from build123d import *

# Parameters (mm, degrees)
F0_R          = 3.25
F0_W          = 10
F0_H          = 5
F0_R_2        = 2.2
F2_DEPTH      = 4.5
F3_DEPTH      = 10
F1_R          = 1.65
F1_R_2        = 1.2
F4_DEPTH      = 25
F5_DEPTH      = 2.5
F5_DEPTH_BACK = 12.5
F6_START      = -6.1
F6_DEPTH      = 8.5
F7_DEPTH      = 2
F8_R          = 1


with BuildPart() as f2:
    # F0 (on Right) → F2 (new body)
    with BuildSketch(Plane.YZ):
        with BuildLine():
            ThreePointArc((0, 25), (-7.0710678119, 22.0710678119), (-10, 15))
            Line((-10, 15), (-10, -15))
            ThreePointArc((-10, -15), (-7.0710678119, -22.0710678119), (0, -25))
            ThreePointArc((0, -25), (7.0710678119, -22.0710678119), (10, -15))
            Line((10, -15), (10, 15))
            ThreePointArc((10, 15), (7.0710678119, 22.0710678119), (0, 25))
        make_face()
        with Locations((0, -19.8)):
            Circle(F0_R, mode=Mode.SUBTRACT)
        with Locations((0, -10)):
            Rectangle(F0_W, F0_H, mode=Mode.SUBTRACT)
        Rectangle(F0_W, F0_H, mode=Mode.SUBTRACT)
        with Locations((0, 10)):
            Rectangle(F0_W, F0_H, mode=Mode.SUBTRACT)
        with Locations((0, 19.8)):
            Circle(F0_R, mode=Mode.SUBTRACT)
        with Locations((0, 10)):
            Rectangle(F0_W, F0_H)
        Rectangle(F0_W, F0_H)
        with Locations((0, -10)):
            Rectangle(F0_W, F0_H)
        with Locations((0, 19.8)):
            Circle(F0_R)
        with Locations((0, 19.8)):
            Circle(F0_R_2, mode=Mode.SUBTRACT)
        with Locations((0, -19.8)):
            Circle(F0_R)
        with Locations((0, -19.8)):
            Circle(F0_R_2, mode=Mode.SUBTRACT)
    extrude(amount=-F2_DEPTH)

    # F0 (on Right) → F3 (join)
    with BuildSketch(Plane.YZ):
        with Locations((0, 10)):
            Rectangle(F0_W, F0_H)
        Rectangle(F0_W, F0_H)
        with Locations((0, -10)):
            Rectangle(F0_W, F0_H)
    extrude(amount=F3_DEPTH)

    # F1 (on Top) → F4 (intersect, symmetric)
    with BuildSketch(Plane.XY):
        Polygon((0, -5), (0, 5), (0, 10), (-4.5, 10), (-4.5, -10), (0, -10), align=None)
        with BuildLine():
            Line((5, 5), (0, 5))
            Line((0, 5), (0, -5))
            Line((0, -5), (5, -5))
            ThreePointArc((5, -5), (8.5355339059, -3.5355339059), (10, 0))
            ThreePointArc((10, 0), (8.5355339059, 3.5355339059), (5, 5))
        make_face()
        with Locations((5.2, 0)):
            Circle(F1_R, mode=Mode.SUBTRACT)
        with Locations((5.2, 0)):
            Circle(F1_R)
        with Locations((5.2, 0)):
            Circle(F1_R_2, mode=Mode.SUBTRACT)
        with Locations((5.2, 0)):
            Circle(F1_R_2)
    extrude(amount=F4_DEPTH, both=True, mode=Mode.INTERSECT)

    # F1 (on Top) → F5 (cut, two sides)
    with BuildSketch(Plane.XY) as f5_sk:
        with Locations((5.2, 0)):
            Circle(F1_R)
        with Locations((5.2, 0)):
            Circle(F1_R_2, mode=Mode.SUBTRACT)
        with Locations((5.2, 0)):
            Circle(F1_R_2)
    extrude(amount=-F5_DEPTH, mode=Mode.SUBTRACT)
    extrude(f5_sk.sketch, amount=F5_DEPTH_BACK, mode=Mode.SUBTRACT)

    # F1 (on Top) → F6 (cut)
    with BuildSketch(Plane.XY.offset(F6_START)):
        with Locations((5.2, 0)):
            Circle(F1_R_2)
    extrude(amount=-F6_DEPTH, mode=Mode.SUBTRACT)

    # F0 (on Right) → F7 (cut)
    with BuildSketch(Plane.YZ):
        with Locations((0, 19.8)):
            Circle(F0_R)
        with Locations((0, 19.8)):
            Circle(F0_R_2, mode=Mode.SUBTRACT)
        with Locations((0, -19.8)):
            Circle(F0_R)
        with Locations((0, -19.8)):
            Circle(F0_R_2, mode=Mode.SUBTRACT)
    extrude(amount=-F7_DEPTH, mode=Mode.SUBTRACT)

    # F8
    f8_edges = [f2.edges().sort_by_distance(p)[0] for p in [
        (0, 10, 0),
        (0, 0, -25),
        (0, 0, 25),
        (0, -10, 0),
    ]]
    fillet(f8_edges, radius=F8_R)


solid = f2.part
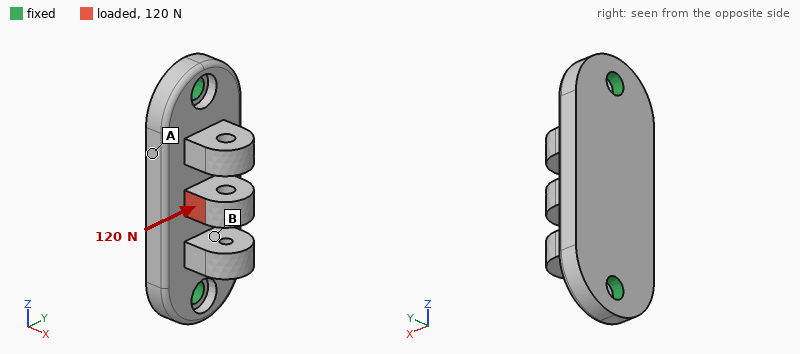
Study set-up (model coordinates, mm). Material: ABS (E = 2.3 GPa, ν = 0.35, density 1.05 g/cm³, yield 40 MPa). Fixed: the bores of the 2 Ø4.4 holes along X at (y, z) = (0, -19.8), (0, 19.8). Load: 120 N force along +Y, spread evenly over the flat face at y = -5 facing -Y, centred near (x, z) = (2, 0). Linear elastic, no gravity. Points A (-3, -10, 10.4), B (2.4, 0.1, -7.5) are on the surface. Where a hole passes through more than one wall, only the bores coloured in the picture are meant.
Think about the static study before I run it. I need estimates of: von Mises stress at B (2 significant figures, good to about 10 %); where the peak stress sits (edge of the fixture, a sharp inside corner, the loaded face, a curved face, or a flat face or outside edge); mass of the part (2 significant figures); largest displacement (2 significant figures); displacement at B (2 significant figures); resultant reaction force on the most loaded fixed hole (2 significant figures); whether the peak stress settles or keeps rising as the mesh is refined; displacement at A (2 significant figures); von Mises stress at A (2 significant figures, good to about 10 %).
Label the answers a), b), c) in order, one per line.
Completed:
a) 1.3 MPa
b) edge of the fixture
c) 5.4 g
d) 0.22 mm
e) 0.076 mm
f) 60 N
g) keeps rising
h) 0.10 mm
i) 2.3 MPa
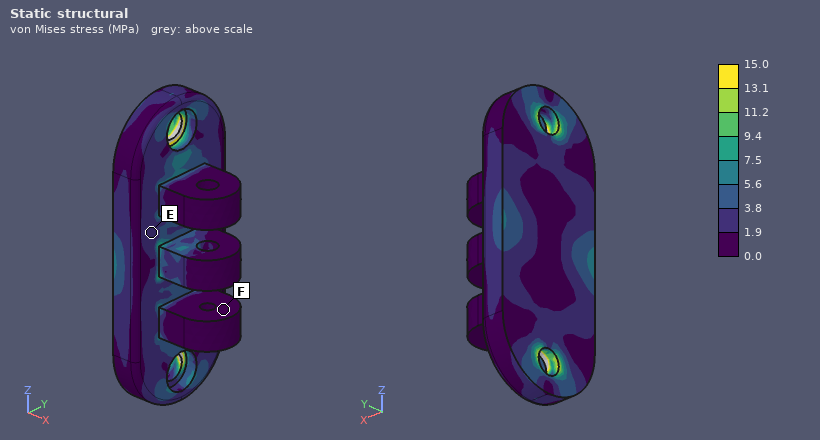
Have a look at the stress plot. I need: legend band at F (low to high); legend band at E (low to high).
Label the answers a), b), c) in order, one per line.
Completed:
a) 0.0 to 1.9 MPa
b) 1.9 to 3.8 MPa
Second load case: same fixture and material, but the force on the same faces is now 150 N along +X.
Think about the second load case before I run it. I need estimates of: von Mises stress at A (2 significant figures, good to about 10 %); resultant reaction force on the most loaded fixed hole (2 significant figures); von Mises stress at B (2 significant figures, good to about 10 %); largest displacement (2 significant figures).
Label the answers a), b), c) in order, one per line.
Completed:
a) 4.6 MPa
b) 110 N
c) 1.9 MPa
d) 0.36 mm
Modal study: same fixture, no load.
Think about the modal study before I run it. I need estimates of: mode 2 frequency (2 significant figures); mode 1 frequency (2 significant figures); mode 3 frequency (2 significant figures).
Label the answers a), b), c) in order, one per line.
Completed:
a) 2700 Hz
b) 2700 Hz
c) 6300 Hz
